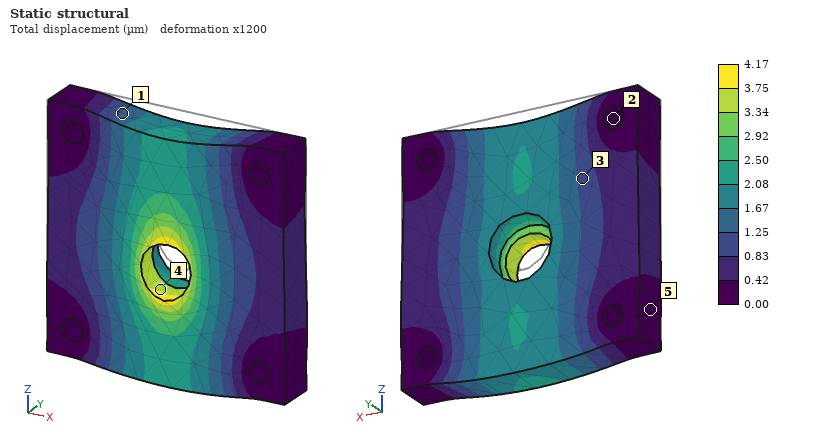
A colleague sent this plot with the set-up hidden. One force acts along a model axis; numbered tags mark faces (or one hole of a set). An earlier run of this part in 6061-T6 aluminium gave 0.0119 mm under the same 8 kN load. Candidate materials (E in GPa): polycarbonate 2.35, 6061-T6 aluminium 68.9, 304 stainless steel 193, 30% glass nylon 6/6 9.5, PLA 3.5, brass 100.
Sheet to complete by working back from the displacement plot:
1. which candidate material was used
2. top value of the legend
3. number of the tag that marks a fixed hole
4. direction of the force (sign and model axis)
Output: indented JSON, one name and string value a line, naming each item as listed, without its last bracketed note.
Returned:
{
  "which candidate material was used": "304 stainless steel",
  "top value of the legend": "4.17 µm",
  "number of the tag that marks a fixed hole": "2",
  "direction of the force": "-Z"
}
